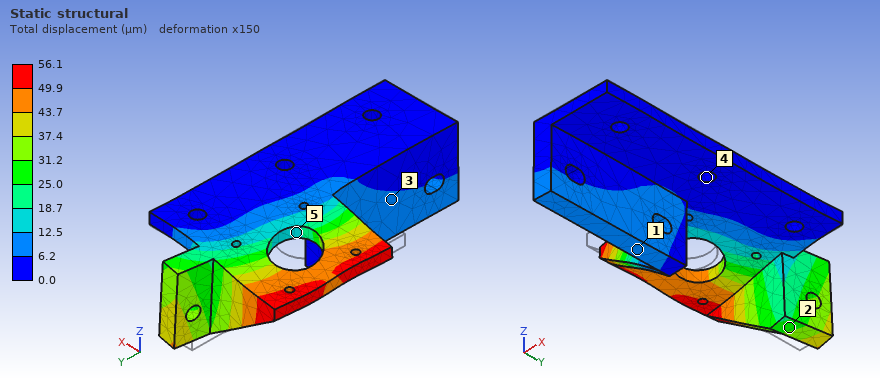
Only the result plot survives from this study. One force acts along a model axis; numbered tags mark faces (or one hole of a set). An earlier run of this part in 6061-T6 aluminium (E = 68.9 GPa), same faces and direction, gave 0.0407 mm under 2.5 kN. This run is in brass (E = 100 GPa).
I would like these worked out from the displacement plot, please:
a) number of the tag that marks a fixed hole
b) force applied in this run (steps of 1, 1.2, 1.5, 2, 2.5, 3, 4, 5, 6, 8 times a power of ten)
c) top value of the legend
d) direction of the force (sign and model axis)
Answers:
4
5 kN
56.1 µm
+Y
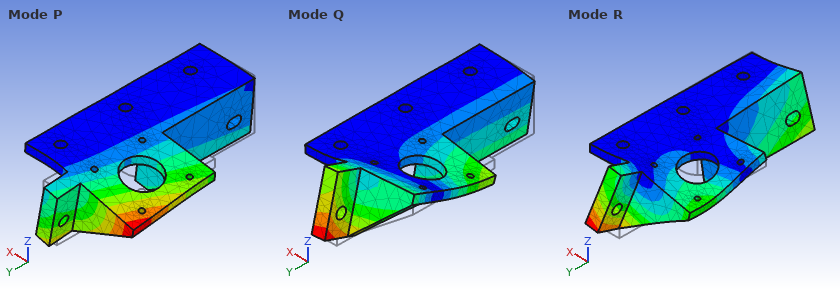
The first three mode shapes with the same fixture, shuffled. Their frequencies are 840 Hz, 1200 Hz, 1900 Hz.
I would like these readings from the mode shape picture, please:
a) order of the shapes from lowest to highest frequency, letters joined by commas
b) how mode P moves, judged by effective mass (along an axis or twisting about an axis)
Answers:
P, Q, R
along Z
